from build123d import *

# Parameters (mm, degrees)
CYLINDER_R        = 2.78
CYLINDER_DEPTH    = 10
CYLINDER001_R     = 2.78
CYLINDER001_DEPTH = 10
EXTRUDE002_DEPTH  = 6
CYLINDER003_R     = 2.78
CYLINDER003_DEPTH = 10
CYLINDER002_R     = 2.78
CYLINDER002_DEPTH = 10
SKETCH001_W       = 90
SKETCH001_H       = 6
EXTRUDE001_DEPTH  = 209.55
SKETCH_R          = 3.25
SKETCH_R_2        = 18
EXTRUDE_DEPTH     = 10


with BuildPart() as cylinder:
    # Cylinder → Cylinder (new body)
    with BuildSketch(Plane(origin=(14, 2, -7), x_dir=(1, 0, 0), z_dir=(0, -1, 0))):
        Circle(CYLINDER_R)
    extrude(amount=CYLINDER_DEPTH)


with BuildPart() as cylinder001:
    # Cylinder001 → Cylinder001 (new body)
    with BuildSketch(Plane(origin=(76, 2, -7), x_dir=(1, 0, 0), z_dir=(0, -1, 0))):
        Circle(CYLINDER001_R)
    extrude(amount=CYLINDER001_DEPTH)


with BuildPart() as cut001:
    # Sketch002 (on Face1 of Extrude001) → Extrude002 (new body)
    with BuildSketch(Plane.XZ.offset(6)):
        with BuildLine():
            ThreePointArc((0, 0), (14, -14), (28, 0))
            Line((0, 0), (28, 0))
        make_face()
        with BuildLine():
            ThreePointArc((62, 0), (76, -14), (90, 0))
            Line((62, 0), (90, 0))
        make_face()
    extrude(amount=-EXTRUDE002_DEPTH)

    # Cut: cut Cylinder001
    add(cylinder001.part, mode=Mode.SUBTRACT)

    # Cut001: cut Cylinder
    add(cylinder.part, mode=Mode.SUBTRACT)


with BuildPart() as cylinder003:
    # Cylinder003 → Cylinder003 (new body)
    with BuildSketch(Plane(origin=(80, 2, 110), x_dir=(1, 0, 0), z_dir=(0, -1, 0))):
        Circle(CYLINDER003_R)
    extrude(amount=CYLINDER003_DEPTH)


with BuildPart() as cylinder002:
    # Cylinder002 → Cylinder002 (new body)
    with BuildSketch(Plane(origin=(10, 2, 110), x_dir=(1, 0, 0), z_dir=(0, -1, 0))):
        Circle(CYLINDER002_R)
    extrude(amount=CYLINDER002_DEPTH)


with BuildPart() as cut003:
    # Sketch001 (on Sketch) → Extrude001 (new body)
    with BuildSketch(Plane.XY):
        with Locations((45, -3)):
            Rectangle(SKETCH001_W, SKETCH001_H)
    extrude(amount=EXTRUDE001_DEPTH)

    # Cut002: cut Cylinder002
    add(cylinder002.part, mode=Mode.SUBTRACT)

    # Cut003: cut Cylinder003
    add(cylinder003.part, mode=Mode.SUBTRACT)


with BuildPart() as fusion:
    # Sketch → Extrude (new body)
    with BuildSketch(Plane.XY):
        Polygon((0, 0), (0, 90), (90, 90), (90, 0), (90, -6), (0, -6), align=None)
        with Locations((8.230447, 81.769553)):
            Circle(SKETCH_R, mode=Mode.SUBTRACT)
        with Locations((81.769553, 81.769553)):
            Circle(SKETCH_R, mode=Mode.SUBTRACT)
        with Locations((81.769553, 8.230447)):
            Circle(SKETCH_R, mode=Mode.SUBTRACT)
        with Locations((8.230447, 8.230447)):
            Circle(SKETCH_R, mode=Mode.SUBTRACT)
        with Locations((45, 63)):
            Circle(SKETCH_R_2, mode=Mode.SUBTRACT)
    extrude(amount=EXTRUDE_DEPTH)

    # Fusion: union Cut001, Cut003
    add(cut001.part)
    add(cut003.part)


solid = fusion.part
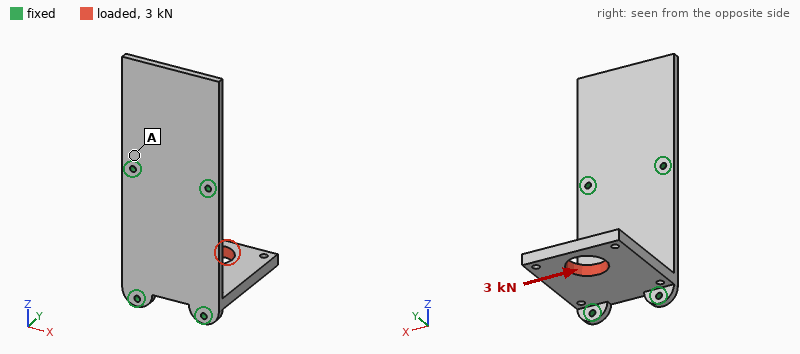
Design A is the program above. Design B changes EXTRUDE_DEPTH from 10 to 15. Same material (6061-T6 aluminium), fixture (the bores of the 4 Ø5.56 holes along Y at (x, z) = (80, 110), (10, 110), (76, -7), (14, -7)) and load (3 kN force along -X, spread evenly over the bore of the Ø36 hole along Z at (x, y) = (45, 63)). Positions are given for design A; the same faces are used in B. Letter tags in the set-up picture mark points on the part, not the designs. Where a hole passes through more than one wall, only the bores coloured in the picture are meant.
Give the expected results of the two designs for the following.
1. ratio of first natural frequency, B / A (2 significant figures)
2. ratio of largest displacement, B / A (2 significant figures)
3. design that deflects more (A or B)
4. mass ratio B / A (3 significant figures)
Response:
1.00
0.84
A
1.19
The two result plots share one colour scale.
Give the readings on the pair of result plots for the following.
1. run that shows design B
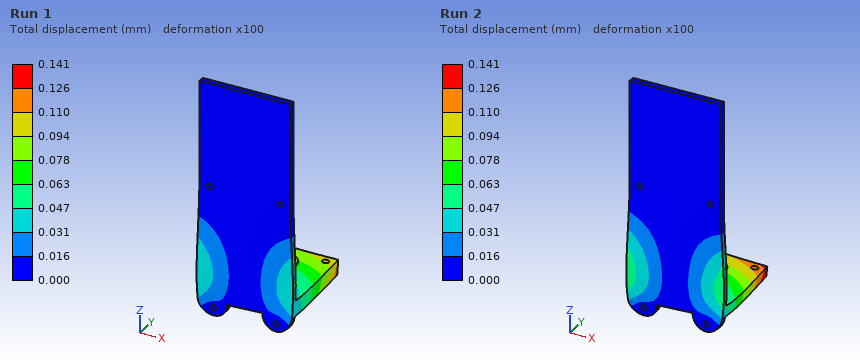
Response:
Run 1
